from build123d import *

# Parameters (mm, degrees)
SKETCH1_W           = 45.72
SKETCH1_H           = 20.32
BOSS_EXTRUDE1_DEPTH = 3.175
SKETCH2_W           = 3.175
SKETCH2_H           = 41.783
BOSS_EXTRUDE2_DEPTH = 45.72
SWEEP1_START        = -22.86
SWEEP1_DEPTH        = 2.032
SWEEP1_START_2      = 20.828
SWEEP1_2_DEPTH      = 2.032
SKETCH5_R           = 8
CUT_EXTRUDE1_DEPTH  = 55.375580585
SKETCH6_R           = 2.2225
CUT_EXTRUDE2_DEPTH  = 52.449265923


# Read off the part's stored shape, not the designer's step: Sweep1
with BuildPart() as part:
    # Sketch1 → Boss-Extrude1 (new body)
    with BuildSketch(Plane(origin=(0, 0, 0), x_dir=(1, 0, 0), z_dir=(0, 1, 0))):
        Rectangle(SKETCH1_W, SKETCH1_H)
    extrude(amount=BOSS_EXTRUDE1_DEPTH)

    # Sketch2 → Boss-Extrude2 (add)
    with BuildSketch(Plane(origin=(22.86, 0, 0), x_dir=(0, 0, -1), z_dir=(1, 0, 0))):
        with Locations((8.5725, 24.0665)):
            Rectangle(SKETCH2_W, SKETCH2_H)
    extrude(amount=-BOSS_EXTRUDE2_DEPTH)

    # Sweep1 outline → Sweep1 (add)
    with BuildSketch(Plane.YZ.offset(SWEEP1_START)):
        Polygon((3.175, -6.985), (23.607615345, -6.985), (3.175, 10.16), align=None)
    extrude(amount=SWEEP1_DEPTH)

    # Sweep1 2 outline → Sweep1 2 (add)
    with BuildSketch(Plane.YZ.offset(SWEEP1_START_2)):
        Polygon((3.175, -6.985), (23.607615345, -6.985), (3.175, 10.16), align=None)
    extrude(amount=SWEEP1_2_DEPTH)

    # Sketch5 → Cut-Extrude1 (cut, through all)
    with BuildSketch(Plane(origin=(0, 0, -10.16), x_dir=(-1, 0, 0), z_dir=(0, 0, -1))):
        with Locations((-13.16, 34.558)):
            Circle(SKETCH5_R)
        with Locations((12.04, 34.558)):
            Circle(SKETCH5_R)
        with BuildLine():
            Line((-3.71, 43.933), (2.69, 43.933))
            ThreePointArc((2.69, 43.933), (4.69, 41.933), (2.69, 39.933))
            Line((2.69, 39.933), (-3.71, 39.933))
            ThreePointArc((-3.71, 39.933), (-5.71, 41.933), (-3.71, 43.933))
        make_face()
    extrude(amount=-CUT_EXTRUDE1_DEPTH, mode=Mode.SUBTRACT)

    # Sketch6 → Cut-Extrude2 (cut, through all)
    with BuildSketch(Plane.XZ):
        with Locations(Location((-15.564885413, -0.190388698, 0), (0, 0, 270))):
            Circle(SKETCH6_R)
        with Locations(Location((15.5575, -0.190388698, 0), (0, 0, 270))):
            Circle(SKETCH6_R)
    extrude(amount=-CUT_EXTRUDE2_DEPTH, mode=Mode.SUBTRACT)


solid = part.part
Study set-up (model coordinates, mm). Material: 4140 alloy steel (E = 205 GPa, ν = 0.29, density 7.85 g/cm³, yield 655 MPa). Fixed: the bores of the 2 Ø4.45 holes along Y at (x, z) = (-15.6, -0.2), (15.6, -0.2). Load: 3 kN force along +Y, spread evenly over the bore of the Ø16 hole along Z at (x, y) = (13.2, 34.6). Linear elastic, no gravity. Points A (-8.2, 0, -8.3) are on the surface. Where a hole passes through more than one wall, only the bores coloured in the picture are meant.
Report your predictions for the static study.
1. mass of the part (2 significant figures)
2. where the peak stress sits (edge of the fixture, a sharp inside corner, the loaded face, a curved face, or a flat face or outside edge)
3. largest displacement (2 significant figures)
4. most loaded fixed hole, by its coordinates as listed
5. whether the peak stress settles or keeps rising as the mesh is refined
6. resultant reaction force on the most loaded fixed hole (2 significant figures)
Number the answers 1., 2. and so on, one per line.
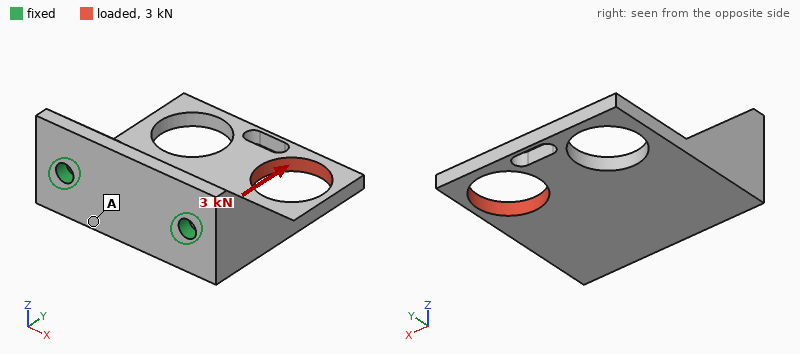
1. 65 g
2. edge of the fixture
3. 0.17 mm
4. (15.6, -0.2)
5. keeps rising
6. 2.6 kN
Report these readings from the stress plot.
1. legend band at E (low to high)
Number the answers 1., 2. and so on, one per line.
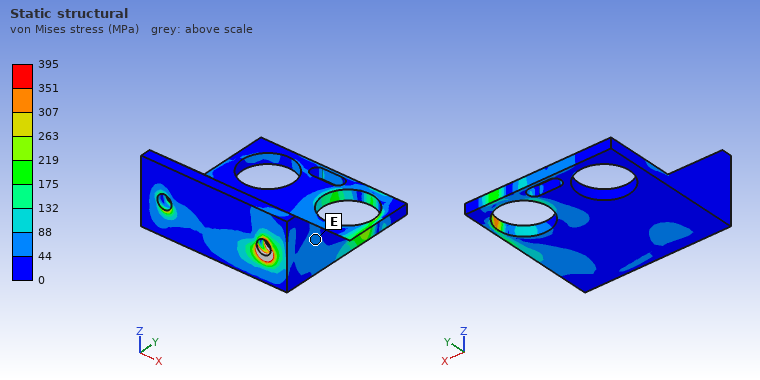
1. 44 to 88 MPa
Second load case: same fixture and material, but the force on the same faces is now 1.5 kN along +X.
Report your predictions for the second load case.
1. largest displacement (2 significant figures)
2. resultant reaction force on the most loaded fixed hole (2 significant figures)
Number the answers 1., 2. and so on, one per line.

1. 90 µm
2. 1.6 kN
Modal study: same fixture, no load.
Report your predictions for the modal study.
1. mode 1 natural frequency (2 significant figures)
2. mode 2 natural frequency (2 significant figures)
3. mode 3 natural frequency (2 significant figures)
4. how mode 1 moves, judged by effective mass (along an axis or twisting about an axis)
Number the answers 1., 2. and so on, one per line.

1. 2200 Hz
2. 4100 Hz
3. 6700 Hz
4. along Z
